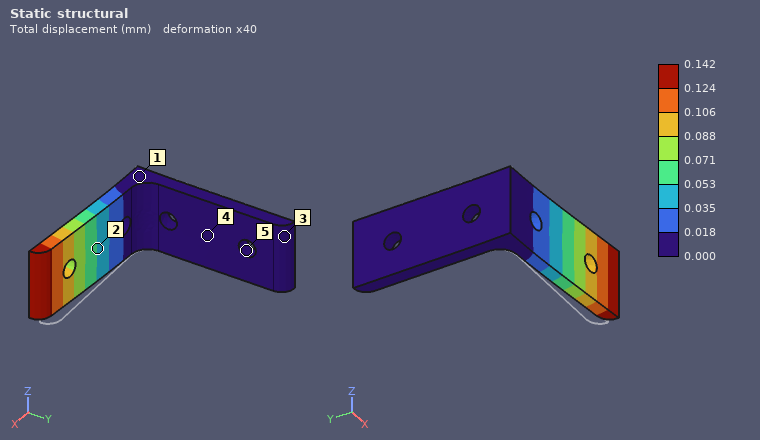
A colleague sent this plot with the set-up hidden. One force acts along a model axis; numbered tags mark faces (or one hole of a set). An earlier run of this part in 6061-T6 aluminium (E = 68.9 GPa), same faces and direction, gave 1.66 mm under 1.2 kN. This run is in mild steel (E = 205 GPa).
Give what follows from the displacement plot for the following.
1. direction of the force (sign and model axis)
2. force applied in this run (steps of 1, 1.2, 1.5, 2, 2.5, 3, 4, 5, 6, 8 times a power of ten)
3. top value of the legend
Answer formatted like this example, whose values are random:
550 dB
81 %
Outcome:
-Y
300 N
0.142 mm
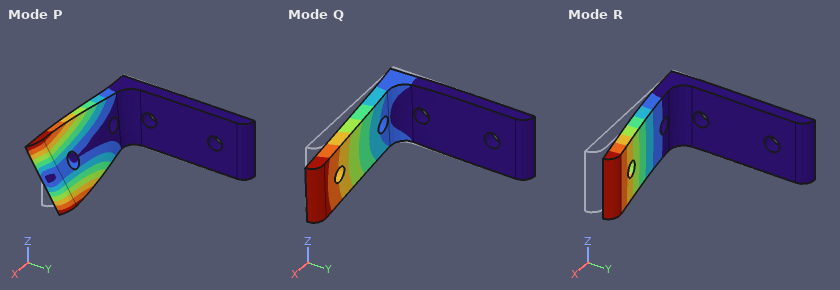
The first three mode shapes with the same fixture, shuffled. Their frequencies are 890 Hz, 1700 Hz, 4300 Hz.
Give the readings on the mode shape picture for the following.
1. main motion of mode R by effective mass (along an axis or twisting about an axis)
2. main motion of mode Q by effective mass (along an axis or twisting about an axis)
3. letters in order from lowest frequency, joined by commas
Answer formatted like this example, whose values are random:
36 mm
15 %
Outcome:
along Y
along Z
R, Q, P
